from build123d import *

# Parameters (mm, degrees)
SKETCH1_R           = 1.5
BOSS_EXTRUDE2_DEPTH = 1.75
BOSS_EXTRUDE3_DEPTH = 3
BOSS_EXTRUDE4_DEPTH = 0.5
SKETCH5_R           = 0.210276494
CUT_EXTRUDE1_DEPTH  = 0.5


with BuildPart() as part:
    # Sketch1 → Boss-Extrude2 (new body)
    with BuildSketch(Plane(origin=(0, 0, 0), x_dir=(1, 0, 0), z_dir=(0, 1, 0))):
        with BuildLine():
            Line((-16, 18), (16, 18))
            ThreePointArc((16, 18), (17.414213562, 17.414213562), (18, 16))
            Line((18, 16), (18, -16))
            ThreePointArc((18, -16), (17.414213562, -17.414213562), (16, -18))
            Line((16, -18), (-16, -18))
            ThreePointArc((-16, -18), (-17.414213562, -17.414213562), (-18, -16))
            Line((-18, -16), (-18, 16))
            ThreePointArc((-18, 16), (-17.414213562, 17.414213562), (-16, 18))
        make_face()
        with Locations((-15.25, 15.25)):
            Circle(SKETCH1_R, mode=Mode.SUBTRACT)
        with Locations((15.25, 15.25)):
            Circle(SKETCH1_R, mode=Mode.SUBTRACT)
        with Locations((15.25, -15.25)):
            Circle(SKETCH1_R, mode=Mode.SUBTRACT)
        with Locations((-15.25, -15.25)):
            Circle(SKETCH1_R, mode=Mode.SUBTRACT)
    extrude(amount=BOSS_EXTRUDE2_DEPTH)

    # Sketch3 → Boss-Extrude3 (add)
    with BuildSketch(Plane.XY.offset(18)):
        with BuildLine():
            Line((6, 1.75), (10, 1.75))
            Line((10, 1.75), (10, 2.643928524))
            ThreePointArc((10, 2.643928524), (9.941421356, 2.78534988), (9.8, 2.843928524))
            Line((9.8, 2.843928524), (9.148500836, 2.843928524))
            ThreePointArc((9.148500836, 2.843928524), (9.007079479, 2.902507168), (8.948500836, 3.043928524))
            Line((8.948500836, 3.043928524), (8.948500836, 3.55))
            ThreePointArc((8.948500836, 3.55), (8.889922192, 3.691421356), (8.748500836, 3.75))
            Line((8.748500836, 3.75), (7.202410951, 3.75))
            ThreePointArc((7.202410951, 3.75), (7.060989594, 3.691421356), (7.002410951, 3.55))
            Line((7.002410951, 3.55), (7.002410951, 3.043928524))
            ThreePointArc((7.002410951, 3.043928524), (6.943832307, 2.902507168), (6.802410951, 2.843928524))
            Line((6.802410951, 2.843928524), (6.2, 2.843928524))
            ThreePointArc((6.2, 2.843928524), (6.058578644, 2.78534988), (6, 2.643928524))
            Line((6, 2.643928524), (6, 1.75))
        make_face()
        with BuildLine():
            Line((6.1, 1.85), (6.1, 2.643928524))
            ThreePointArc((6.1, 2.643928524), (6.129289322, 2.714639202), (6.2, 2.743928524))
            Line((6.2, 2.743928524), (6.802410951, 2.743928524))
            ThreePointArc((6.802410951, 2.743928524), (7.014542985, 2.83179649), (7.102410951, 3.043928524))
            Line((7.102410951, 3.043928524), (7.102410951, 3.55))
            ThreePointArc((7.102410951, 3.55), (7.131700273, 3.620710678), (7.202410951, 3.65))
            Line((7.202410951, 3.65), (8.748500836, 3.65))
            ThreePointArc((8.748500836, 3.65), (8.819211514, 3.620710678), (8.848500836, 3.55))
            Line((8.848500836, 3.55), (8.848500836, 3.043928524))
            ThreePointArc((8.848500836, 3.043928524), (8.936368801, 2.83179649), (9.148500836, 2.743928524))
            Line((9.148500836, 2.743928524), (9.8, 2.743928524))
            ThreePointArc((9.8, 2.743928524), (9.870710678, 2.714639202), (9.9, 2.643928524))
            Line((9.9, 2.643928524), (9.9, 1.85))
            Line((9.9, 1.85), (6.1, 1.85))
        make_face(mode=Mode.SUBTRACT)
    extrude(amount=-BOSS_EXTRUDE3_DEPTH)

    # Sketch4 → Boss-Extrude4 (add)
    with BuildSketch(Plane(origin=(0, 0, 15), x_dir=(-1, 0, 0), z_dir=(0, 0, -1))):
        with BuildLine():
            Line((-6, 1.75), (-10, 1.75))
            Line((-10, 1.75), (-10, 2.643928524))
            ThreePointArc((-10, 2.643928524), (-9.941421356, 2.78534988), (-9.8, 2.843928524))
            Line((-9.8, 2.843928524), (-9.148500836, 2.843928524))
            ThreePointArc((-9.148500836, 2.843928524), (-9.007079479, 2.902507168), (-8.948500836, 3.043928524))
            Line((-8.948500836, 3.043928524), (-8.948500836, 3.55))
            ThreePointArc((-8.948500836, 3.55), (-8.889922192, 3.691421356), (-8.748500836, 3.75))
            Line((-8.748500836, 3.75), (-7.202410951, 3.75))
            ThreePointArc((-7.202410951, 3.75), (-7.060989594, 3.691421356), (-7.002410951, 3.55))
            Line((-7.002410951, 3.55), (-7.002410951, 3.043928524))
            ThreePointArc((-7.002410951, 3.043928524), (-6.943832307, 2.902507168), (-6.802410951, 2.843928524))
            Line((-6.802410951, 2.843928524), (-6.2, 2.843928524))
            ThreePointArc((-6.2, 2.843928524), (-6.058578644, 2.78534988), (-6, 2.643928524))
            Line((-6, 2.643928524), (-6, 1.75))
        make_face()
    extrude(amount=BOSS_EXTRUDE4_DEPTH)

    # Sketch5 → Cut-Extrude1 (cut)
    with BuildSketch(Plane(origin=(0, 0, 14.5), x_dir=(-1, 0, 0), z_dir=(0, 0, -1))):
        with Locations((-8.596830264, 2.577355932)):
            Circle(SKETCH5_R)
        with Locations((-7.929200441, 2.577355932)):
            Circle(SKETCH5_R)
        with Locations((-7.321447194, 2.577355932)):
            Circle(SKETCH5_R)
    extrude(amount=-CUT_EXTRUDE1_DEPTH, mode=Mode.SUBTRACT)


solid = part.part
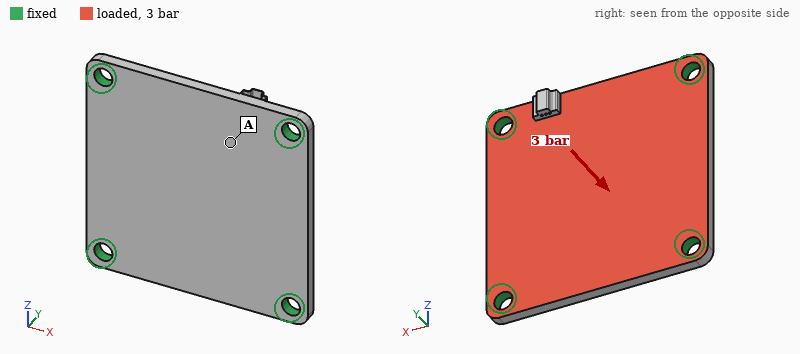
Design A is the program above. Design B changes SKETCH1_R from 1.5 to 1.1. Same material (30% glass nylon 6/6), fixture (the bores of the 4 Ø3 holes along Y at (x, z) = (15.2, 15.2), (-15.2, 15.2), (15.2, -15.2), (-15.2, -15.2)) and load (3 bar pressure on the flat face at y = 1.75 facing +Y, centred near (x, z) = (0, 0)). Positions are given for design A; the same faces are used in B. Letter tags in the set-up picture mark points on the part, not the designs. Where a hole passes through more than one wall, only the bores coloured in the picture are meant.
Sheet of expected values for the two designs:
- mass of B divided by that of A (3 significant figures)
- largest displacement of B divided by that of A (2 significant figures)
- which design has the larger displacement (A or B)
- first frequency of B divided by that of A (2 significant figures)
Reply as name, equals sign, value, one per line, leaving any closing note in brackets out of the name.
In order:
mass of B divided by that of A = 1.01
largest displacement of B divided by that of A = 1.1
which design has the larger displacement = B
first frequency of B divided by that of A = 0.93
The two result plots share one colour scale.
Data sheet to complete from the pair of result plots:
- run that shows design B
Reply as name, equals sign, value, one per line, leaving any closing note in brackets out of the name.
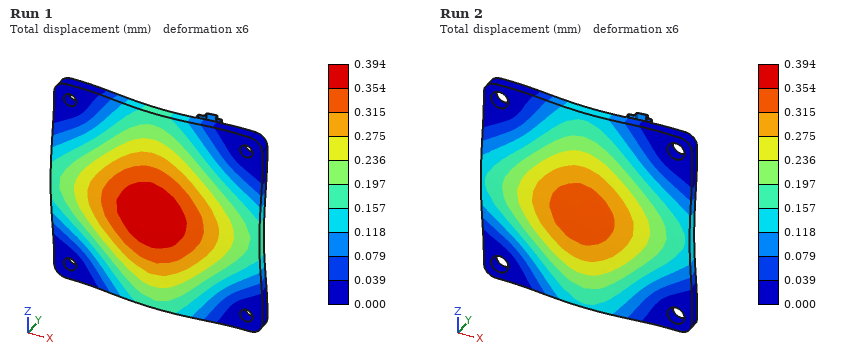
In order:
run that shows design B = Run 1
